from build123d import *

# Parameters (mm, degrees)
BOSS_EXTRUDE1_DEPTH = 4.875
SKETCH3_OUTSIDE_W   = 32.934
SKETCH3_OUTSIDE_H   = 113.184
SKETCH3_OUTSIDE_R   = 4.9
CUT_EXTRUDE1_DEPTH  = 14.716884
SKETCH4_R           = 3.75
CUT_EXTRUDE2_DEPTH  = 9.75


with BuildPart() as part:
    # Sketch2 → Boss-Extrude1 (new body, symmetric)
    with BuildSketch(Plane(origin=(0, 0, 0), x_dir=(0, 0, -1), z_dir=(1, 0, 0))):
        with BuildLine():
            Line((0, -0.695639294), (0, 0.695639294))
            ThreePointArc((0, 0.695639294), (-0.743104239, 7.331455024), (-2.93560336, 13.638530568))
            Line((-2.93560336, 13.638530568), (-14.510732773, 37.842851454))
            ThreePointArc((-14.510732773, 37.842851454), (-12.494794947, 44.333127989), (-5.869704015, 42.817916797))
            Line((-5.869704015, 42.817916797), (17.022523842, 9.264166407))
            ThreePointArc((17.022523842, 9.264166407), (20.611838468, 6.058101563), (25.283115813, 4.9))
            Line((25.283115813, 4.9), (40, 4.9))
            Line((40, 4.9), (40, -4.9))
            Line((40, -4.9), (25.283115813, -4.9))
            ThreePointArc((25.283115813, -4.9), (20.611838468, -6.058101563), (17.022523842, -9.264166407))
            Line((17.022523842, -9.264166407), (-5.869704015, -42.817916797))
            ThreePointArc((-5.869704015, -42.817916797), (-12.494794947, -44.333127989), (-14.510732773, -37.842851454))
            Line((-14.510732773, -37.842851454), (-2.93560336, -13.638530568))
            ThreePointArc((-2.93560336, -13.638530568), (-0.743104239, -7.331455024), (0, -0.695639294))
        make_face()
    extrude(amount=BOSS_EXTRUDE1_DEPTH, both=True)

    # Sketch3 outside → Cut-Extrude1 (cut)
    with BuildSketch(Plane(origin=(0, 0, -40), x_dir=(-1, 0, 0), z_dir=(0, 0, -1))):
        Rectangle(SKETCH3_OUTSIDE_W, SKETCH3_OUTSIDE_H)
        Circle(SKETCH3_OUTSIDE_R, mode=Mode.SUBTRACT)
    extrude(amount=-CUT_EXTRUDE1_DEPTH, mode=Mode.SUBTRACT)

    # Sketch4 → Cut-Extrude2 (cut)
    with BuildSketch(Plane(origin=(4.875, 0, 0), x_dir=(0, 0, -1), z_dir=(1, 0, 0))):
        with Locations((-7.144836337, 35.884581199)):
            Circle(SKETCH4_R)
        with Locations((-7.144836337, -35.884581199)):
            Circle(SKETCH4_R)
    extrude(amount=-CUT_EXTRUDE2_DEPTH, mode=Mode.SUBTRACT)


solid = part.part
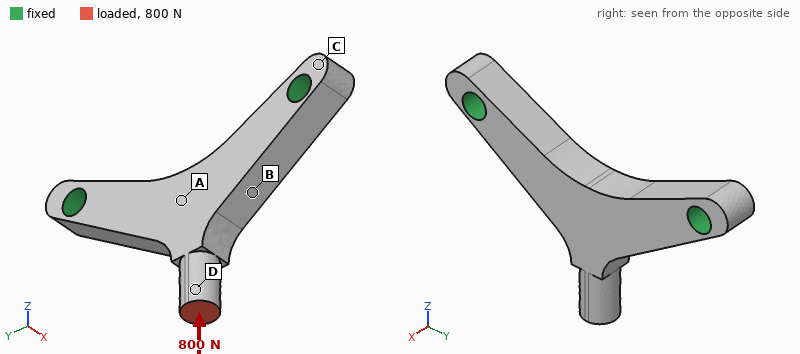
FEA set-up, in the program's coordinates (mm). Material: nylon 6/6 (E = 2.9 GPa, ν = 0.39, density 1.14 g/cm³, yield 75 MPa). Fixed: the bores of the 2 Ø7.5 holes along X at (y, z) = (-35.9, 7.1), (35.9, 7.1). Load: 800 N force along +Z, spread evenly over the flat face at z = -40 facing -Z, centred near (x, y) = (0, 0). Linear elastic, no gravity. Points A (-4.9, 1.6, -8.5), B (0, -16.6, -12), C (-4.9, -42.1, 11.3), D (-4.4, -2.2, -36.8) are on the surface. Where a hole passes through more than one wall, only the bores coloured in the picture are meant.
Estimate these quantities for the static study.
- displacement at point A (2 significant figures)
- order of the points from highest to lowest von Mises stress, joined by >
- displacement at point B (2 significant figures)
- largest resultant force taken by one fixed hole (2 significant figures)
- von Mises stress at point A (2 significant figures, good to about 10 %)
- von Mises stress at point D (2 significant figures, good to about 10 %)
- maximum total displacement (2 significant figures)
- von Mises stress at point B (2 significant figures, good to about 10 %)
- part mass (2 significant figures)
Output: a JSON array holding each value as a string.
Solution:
["0.12 mm", "D > B > A > C", "0.081 mm", "630 N", "2.3 MPa", "11 MPa", "0.19 mm", "7.4 MPa", "16 g"]
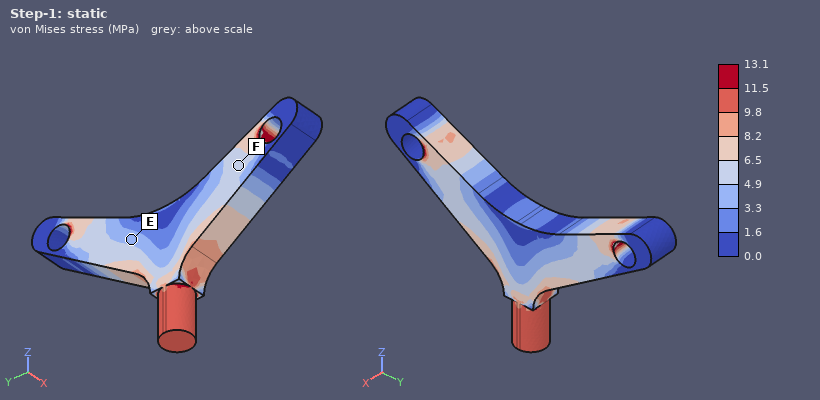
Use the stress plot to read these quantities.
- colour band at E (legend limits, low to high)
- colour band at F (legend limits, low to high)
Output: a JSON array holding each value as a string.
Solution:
["3.3 to 4.9 MPa", "4.9 to 6.5 MPa"]
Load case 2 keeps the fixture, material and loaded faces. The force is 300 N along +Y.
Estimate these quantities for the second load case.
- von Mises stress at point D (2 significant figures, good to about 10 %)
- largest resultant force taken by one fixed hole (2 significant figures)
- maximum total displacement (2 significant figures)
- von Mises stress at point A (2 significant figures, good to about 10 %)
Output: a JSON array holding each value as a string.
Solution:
["9.0 MPa", "280 N", "0.81 mm", "5.2 MPa"]
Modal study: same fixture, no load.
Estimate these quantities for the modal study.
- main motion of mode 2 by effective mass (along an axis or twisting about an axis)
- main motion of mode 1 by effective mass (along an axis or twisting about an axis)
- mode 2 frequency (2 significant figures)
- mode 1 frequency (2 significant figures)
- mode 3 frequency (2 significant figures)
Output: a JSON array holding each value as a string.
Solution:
["along X", "along X", "3400 Hz", "1200 Hz", "4100 Hz"]
